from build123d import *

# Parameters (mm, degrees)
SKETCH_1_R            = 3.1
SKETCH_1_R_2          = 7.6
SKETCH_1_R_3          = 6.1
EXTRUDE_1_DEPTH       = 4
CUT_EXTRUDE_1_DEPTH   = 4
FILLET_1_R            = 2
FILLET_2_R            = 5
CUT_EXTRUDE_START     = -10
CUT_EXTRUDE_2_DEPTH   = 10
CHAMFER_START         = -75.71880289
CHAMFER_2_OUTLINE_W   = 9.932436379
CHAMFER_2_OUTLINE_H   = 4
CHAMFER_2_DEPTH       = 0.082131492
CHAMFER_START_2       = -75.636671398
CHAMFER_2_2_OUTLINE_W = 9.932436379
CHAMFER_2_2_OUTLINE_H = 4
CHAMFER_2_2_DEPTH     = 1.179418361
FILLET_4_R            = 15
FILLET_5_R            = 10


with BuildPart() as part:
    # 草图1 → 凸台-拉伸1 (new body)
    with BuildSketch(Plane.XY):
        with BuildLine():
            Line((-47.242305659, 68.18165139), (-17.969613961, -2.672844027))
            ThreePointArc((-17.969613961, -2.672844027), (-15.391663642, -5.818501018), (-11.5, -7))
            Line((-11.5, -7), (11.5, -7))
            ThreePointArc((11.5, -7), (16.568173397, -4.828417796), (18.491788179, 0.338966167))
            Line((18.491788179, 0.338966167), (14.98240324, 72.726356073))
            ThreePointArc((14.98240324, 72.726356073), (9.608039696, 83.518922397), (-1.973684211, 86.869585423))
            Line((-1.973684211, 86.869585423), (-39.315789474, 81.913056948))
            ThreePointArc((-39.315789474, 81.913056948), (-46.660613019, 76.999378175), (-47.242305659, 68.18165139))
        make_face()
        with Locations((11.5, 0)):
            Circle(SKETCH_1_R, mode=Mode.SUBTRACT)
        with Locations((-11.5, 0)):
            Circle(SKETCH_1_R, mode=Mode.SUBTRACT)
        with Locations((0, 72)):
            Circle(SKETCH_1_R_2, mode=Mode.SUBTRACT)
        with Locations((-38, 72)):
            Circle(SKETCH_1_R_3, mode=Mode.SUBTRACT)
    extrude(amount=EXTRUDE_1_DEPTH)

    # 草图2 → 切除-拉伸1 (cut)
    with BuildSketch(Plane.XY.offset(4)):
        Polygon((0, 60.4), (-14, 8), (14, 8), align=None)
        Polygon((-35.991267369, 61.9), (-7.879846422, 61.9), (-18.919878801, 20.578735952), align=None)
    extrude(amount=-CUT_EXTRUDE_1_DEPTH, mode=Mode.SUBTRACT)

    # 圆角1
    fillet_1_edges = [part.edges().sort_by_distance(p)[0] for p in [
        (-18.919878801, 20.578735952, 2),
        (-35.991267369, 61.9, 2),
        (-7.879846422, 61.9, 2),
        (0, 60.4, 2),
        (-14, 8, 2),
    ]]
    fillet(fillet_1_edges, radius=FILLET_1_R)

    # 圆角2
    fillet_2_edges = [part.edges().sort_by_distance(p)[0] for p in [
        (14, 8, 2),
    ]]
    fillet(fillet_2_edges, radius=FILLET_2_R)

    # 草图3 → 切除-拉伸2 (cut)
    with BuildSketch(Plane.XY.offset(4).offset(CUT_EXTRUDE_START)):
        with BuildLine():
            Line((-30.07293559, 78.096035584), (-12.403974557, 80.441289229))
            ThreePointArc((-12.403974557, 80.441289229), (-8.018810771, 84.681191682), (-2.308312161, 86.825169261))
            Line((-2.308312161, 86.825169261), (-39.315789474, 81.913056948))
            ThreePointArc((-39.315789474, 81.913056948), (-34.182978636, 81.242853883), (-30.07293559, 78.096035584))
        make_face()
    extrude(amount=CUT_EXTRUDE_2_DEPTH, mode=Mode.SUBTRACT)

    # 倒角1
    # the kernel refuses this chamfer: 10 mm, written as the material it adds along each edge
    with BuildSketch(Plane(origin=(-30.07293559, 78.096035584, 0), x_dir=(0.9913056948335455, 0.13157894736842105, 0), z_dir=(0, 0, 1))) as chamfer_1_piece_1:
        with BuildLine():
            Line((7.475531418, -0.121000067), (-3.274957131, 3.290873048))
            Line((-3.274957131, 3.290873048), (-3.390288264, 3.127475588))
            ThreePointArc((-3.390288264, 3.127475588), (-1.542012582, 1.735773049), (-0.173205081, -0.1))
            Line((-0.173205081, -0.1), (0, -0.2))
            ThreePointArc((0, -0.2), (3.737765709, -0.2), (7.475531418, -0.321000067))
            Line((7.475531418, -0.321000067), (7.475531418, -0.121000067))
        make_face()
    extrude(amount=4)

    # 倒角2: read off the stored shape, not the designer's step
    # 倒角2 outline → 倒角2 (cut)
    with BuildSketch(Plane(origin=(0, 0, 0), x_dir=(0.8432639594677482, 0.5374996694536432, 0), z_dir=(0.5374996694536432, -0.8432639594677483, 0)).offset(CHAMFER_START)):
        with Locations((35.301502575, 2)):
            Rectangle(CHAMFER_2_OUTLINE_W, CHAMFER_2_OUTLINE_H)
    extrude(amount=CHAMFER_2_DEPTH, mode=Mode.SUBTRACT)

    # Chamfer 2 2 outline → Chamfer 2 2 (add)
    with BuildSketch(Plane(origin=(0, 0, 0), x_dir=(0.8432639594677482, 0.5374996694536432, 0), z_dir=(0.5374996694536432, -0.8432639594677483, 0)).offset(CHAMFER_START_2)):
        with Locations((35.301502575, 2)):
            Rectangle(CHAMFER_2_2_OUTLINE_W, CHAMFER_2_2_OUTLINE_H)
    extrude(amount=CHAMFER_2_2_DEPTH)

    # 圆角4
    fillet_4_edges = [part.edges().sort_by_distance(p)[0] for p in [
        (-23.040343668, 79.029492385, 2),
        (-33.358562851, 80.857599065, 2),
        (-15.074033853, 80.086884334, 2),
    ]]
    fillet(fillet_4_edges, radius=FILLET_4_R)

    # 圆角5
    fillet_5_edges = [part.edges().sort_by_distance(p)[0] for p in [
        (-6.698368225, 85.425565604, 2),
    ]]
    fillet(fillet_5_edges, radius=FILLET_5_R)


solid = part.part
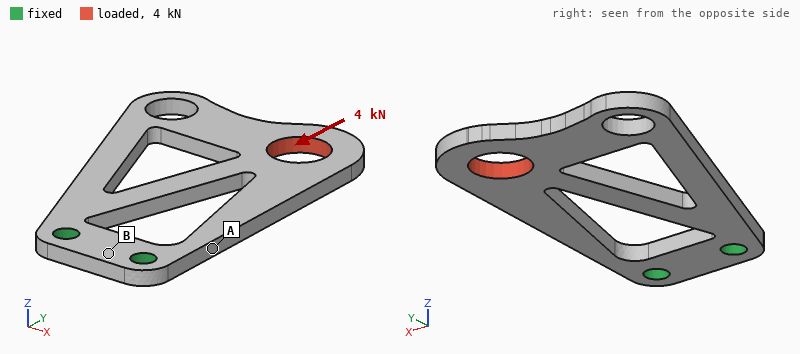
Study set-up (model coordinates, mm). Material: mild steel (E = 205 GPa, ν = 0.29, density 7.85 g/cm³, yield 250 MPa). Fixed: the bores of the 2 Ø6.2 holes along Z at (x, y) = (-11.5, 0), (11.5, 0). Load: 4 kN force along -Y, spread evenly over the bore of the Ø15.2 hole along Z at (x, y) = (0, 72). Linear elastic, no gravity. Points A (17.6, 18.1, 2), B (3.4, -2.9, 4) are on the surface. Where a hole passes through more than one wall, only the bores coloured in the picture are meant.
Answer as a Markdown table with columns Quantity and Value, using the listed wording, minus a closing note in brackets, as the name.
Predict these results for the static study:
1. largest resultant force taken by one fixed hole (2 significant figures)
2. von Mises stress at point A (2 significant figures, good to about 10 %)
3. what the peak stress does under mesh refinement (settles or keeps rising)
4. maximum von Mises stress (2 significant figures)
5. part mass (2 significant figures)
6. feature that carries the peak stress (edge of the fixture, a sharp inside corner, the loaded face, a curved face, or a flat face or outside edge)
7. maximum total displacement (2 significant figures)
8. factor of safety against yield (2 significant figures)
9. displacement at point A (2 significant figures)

| Quantity | Value |
|---|---|
| largest resultant force taken by one fixed hole | 2.1 kN |
| von Mises stress at point A | 44 MPa |
| what the peak stress does under mesh refinement | settles |
| maximum von Mises stress | 190 MPa |
| part mass | 90 g |
| feature that carries the peak stress | a curved face |
| maximum total displacement | 28 µm |
| factor of safety against yield | 1.3 |
| displacement at point A | 11 µm |
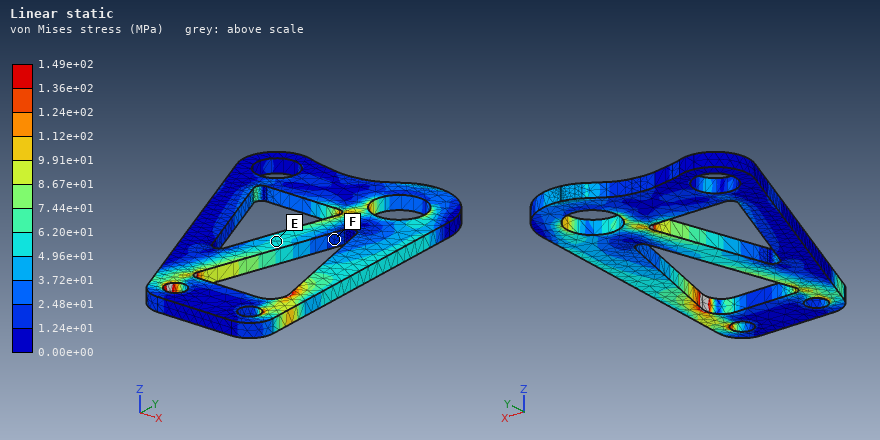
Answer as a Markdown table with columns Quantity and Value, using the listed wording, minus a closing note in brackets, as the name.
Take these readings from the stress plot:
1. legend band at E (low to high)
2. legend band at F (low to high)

| Quantity | Value |
|---|---|
| legend band at E | 4.96e+01 to 6.20e+01 MPa |
| legend band at F | 1.24e+01 to 2.48e+01 MPa |
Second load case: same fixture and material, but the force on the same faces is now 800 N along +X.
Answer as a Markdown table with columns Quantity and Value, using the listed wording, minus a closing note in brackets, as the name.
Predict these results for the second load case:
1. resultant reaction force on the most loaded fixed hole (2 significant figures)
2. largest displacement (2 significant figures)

| Quantity | Value |
|---|---|
| resultant reaction force on the most loaded fixed hole | 1.8 kN |
| largest displacement | 92 µm |
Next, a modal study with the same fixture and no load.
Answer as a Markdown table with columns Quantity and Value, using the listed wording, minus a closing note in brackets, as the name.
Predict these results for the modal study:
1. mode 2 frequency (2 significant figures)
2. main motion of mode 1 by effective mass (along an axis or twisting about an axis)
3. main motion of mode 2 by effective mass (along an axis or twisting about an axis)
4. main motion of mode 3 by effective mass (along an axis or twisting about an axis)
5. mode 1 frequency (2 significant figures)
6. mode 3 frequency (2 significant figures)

| Quantity | Value |
|---|---|
| mode 2 frequency | 990 Hz |
| main motion of mode 1 by effective mass | along Z |
| main motion of mode 2 by effective mass | twisting about Y |
| main motion of mode 3 by effective mass | along X |
| mode 1 frequency | 340 Hz |
| mode 3 frequency | 2300 Hz |
